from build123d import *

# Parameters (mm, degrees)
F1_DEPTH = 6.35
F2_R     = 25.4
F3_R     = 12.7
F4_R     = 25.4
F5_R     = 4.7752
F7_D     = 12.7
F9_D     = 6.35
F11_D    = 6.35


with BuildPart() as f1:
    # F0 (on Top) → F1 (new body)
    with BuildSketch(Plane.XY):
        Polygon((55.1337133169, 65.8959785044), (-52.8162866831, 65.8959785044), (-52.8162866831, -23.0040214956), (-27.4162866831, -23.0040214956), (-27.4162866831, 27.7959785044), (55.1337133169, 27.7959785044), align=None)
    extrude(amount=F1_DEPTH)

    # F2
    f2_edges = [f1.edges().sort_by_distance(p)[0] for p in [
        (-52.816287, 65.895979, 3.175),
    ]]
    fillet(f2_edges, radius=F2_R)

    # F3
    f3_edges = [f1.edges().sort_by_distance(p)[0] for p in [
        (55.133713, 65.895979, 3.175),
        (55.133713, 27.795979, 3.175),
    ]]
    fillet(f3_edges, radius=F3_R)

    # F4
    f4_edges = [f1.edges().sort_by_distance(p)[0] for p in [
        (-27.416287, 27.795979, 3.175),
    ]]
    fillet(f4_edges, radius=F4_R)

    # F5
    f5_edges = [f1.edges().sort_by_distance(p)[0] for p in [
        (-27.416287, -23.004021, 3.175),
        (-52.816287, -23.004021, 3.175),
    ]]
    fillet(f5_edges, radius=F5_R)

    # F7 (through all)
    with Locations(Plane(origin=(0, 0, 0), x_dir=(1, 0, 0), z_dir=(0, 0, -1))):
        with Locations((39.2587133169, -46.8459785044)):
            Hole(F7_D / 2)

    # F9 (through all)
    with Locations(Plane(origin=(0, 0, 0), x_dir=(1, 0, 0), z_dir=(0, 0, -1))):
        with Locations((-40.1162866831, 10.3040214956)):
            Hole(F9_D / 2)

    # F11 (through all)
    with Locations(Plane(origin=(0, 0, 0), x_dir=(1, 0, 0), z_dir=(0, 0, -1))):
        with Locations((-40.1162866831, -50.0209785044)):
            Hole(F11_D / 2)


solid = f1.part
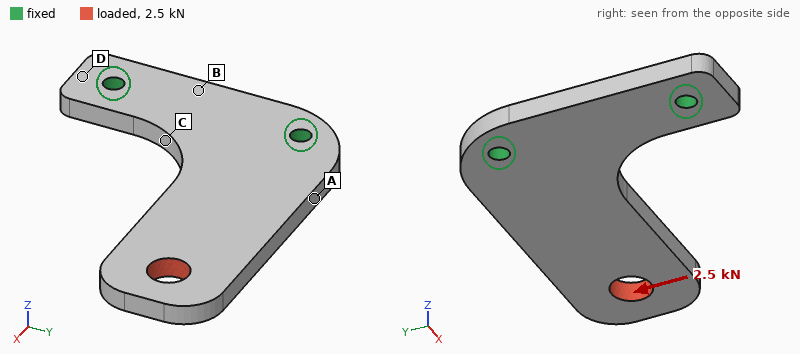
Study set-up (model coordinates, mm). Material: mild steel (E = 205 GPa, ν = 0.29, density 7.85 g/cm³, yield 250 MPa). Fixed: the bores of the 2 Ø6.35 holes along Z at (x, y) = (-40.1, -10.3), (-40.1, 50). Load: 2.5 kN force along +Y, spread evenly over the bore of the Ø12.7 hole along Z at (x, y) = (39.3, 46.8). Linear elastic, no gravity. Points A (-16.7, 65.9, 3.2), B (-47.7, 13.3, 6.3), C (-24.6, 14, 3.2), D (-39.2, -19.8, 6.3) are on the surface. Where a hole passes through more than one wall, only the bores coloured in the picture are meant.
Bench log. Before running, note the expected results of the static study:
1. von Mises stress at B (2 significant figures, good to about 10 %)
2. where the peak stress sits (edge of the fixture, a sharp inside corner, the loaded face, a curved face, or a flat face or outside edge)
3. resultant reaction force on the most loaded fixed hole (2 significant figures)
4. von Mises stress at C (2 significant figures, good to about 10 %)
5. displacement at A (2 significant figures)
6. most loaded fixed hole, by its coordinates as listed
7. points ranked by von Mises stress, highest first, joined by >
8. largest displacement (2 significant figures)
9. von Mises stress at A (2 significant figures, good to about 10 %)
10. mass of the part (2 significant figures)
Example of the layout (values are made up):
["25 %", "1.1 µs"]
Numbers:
["28 MPa", "edge of the fixture", "3.8 kN", "120 MPa", "0.021 mm", "(-40.1, -10.3)", "C > A > B > D", "0.11 mm", "69 MPa", "260 g"]
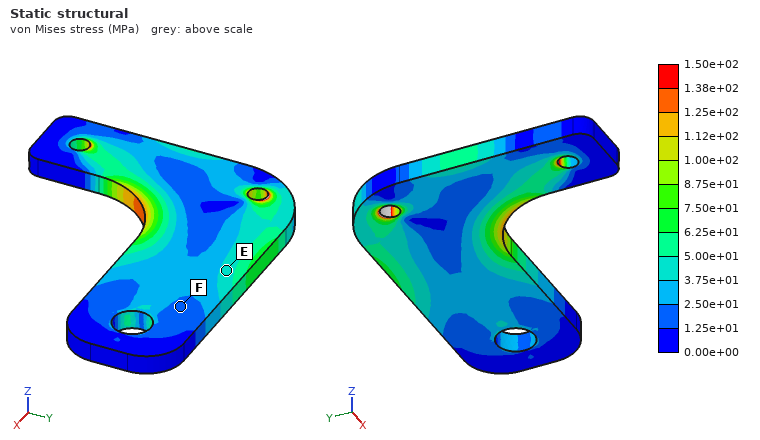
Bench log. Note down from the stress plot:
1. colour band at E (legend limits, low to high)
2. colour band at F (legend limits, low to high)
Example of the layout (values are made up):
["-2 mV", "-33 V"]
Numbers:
["3.75e+01 to 5.00e+01 MPa", "1.25e+01 to 2.50e+01 MPa"]
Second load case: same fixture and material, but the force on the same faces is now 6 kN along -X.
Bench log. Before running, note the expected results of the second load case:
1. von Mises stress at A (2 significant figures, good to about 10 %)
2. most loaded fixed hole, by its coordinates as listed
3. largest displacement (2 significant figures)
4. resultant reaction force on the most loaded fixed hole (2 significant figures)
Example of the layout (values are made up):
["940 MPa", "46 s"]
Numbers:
["24 MPa", "(-40.1, 50)", "15 µm", "5.6 kN"]
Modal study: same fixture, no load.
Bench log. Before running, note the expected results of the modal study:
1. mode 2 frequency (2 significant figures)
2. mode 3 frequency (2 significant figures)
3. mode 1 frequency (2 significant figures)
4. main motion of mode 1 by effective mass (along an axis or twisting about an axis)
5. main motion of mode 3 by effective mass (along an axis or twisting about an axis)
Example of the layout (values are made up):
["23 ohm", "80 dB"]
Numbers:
["3000 Hz", "3300 Hz", "650 Hz", "along Z", "along Y"]
